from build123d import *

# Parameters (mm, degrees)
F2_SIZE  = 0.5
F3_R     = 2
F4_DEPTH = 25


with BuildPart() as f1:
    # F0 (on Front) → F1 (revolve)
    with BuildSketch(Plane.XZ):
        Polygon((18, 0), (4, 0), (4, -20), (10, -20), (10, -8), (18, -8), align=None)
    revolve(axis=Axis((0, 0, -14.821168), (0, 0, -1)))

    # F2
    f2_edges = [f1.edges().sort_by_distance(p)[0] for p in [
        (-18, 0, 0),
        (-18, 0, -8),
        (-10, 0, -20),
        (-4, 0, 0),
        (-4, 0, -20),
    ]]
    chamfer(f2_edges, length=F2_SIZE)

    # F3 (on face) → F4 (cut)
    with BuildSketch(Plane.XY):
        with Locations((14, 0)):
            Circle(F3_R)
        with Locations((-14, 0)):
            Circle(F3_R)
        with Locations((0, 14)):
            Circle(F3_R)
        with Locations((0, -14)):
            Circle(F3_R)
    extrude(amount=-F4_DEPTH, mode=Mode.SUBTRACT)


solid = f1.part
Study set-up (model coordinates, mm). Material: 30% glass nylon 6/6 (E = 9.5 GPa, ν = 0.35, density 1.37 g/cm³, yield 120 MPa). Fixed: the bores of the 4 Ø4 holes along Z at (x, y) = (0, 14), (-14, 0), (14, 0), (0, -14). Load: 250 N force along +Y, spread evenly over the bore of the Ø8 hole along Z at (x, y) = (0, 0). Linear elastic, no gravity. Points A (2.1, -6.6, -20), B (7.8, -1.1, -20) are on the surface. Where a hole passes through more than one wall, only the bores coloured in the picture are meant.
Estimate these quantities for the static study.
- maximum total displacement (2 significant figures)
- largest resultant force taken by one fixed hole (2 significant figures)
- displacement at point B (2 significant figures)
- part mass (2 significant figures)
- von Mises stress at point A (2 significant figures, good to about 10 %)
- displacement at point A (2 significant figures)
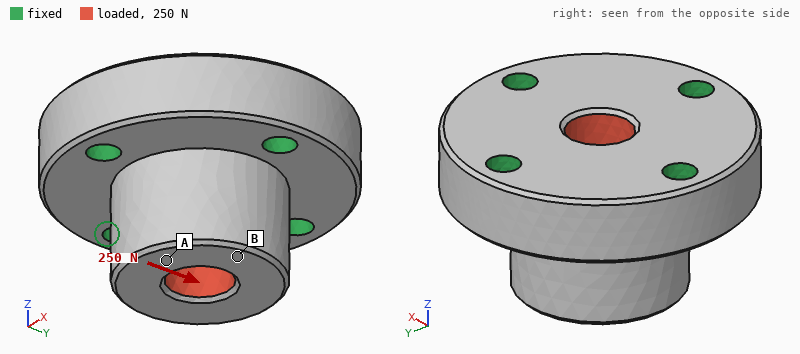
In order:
4.0 µm
97 N
3.4 µm
14 g
0.60 MPa
3.9 µm
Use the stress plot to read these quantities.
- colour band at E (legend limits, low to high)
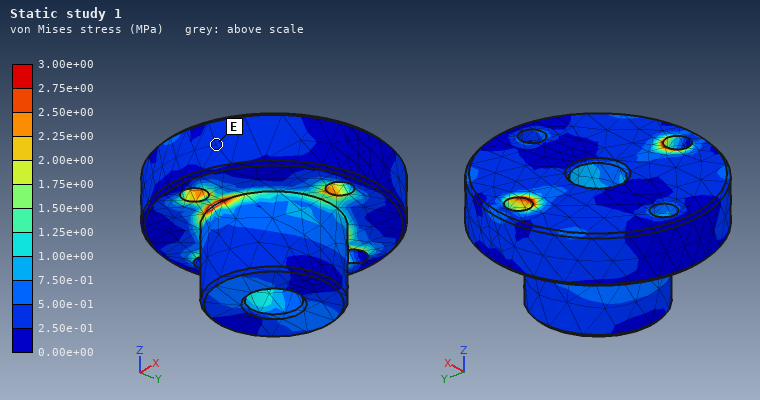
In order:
2.50e-01 to 5.00e-01 MPa
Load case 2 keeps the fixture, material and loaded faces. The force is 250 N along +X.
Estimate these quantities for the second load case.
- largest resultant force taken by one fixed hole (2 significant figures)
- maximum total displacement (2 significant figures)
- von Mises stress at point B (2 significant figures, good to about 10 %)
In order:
97 N
4.0 µm
0.57 MPa
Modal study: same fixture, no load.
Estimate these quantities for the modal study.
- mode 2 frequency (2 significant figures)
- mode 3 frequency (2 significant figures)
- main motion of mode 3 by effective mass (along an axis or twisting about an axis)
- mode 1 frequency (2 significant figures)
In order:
17 kHz
22 kHz
along Z
17 kHz
